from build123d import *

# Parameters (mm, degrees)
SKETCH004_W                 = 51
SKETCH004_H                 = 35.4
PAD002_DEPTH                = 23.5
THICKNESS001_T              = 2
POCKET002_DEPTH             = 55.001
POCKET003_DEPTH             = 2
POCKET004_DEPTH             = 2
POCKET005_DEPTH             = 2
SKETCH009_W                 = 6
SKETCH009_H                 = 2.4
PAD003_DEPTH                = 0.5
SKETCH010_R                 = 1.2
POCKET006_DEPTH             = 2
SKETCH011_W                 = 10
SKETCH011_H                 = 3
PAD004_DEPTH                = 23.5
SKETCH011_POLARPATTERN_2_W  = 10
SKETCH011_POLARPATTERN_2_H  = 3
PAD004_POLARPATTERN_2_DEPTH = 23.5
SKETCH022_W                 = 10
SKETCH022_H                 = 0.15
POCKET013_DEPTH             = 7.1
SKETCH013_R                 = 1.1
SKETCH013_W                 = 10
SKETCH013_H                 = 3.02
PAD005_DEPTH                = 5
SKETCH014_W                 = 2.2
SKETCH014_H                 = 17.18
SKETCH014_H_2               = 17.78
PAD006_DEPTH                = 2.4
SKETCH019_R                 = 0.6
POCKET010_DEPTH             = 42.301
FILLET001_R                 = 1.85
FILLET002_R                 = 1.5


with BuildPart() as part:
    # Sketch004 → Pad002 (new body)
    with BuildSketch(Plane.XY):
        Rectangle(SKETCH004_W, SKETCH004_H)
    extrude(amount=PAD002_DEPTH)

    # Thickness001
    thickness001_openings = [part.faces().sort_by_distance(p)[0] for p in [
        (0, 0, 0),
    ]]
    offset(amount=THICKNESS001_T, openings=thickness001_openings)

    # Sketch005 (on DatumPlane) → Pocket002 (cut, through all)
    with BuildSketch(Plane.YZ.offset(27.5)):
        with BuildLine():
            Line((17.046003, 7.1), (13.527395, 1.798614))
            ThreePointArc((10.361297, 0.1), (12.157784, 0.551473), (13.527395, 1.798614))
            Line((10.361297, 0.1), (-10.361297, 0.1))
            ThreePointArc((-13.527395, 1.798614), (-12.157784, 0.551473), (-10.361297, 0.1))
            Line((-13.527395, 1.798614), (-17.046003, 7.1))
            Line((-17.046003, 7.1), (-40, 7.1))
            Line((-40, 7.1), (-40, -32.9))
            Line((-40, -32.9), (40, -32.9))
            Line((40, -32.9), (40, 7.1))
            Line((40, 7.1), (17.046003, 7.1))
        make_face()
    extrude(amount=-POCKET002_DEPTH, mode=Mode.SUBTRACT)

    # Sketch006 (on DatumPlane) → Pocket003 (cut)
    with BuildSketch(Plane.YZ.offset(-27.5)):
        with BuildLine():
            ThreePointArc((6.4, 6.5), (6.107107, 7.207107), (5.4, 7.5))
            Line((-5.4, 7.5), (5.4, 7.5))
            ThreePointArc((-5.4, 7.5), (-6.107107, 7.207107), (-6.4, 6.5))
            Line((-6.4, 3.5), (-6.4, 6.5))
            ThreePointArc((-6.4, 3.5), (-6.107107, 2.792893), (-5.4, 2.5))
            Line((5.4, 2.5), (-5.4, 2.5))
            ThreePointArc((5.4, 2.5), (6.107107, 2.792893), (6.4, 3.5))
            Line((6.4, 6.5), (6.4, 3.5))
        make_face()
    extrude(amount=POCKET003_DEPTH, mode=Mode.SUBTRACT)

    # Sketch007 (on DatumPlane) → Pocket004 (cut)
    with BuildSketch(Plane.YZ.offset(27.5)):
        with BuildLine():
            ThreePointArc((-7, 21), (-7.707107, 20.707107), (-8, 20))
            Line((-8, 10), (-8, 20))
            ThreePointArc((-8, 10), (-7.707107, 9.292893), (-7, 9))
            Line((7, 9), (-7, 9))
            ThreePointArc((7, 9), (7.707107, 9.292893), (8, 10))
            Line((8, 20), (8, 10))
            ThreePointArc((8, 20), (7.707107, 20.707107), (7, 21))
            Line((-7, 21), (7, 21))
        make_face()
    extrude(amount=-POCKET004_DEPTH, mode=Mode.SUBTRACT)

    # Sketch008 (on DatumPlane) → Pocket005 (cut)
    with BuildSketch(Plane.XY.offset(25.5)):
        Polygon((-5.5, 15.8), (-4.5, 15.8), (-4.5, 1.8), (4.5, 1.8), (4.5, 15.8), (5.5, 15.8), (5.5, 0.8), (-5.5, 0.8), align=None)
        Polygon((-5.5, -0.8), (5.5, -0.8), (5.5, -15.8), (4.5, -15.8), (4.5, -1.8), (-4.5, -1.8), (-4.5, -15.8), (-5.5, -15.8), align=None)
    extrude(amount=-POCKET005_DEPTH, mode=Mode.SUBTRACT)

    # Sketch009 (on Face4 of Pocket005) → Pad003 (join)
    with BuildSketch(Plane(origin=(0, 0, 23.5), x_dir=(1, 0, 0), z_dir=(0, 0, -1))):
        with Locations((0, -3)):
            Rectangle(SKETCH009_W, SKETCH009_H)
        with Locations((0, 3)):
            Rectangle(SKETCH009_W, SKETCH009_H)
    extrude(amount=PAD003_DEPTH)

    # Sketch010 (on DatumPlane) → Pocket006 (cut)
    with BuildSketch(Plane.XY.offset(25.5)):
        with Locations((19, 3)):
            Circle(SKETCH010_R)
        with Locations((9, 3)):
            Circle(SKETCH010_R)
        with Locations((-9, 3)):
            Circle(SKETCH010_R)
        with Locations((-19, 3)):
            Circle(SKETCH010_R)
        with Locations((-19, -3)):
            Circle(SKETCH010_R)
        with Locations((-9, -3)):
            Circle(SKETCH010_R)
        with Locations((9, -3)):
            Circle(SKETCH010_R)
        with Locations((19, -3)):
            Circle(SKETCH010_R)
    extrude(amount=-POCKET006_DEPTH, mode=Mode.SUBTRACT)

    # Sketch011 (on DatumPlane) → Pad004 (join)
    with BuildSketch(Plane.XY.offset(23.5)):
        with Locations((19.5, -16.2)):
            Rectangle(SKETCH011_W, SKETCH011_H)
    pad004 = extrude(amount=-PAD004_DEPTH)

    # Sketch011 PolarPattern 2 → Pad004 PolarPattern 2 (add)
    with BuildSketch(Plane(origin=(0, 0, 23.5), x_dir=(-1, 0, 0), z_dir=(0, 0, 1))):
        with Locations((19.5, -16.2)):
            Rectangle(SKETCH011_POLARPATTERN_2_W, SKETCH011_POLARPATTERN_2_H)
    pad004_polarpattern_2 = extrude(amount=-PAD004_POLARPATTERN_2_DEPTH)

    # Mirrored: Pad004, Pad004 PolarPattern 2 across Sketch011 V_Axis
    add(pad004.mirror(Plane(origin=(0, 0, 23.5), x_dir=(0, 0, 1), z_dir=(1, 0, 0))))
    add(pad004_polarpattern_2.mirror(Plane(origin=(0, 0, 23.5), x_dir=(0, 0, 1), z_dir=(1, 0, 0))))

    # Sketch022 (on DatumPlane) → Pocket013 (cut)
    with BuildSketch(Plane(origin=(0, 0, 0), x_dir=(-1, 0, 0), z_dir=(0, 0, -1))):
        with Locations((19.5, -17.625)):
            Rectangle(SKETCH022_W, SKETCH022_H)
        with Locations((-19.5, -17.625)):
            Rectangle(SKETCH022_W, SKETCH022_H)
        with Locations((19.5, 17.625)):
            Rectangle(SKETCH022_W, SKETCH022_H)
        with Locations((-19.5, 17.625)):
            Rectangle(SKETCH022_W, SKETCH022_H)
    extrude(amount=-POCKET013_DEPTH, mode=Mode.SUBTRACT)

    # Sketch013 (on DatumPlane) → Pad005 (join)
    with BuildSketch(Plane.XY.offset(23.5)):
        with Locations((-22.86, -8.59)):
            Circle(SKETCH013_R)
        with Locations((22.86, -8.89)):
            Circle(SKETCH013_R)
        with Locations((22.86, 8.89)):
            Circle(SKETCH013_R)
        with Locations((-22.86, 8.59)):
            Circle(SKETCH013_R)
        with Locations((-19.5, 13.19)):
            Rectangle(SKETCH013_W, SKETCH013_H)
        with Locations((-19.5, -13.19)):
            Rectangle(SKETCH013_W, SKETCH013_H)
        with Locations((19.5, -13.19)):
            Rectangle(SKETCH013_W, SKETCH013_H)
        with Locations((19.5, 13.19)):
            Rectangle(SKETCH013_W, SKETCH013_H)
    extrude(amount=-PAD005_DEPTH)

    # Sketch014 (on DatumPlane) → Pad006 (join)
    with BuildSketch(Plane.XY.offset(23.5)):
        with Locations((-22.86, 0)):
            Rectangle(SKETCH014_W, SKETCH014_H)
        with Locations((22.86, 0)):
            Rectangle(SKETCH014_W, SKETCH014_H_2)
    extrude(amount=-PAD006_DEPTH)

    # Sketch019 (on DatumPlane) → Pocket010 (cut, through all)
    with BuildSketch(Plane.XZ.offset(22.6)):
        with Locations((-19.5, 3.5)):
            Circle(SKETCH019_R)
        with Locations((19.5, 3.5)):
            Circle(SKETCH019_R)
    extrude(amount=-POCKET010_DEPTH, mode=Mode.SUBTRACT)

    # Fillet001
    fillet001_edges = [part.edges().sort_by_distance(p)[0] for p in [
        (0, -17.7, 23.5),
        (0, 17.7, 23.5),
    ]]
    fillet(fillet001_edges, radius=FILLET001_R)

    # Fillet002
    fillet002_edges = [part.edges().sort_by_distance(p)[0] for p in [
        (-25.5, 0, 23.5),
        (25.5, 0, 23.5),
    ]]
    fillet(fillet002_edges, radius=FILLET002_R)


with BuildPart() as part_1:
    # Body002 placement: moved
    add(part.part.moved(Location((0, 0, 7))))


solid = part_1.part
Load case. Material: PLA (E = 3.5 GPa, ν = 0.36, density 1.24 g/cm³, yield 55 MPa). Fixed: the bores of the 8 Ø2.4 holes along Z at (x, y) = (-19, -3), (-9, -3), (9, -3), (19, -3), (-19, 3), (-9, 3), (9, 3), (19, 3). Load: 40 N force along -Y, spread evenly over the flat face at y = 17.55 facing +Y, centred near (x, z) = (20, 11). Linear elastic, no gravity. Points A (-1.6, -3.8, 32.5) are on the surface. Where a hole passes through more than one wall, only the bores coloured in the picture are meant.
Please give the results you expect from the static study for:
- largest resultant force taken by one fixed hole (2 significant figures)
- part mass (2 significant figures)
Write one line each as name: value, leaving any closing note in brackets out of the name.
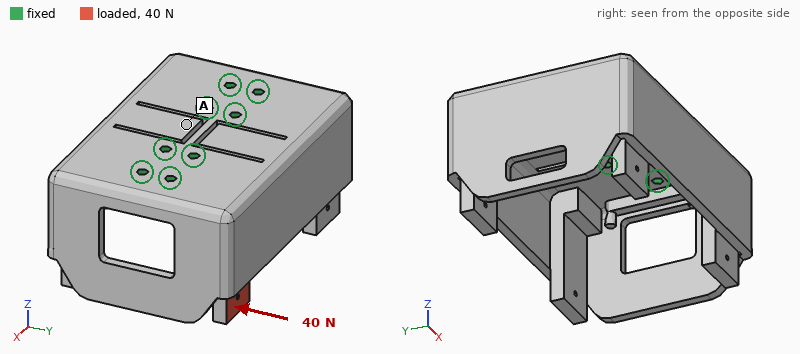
largest resultant force taken by one fixed hole: 62 N
part mass: 17 g
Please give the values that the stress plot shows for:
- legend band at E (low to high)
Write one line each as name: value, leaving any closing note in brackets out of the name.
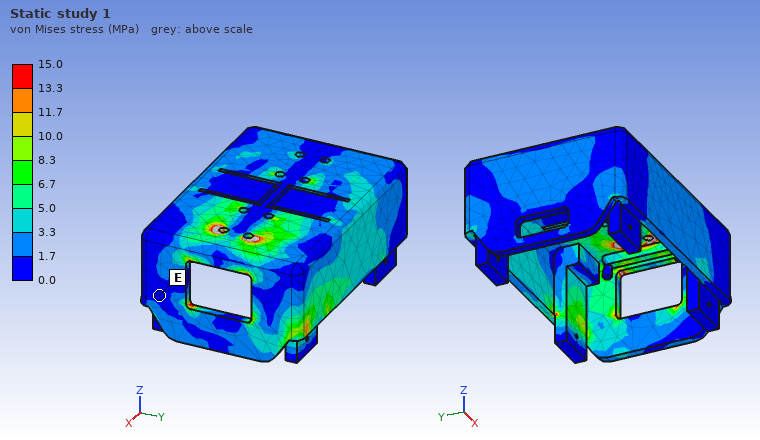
legend band at E: 0.0 to 1.7 MPa
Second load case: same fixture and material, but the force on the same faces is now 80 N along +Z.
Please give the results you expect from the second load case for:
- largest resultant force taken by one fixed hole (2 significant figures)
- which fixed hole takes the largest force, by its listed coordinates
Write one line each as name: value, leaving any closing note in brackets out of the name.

largest resultant force taken by one fixed hole: 120 N
which fixed hole takes the largest force, by its listed coordinates: (19, 3)
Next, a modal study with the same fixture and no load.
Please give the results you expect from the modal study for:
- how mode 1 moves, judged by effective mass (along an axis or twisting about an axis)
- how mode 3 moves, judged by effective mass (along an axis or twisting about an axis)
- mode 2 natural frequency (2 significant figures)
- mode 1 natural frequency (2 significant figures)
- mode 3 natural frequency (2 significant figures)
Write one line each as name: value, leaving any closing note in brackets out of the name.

how mode 1 moves, judged by effective mass: along Y
how mode 3 moves, judged by effective mass: along X
mode 2 natural frequency: 860 Hz
mode 1 natural frequency: 800 Hz
mode 3 natural frequency: 1600 Hz
